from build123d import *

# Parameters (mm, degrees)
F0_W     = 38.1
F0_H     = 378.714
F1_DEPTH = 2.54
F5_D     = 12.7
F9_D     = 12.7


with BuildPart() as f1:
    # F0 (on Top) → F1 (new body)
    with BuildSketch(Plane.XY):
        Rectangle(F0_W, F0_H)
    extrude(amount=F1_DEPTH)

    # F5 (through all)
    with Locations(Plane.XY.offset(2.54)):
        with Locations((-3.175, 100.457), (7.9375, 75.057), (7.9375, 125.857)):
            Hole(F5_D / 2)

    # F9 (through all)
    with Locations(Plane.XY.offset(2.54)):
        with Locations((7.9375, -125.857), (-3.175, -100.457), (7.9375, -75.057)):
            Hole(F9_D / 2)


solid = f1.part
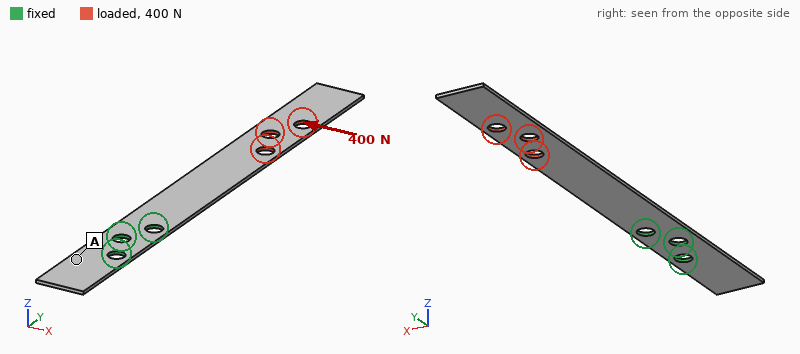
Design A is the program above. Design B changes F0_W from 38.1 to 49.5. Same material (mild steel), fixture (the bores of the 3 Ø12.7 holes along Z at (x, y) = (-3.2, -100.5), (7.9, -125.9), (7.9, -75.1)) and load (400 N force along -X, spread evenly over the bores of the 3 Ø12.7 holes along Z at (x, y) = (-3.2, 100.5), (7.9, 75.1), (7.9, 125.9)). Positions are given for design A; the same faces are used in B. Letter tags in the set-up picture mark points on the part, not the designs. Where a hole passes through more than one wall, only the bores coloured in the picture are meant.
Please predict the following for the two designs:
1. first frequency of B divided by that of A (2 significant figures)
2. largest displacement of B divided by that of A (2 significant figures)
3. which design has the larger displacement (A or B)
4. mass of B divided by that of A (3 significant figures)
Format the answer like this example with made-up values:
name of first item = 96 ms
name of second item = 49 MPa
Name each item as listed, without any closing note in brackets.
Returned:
first frequency of B divided by that of A = 0.99
largest displacement of B divided by that of A = 0.50
which design has the larger displacement = A
mass of B divided by that of A = 1.32
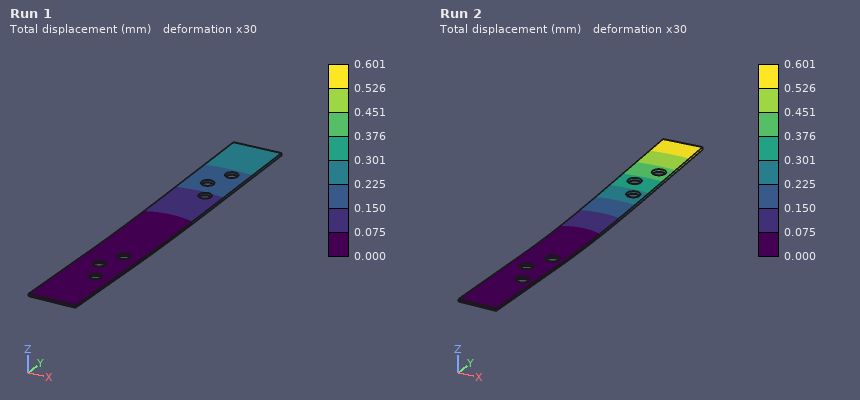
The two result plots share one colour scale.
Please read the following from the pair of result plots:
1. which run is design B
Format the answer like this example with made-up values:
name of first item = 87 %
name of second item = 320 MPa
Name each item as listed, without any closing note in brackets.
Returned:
which run is design B = Run 1
